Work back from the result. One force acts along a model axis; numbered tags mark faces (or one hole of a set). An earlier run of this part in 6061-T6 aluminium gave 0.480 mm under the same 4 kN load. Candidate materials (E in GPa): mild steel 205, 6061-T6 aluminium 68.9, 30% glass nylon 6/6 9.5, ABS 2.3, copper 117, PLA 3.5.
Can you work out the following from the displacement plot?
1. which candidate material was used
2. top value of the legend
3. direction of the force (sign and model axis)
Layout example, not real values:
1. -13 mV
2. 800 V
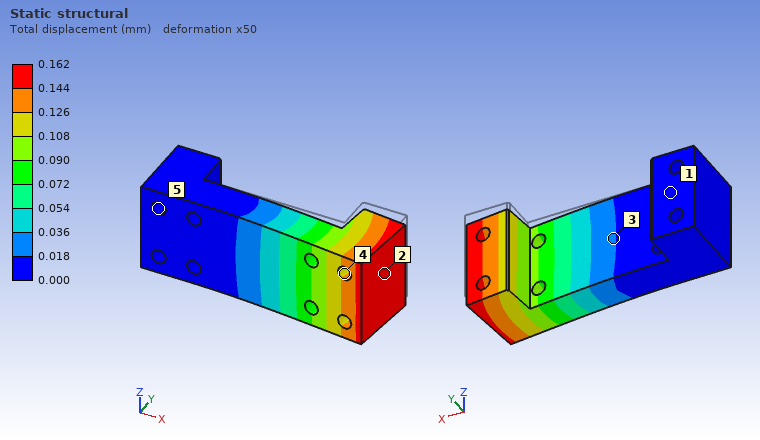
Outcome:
1. mild steel
2. 0.162 mm
3. -Y
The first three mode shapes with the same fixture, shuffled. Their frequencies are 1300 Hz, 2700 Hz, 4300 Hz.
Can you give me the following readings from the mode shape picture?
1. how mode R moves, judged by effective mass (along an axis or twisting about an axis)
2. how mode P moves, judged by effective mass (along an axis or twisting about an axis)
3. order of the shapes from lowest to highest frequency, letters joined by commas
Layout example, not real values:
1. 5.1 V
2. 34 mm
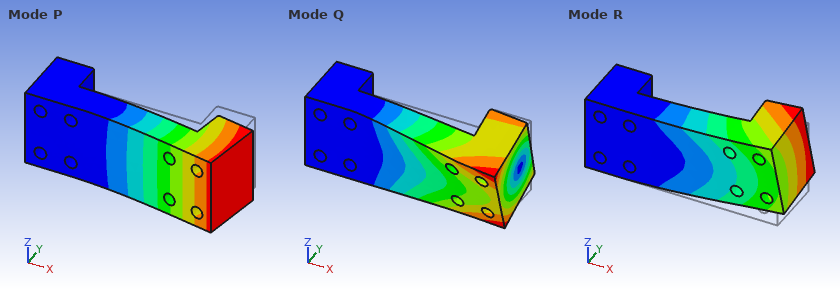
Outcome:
1. along Z
2. along Y
3. P, R, Q
